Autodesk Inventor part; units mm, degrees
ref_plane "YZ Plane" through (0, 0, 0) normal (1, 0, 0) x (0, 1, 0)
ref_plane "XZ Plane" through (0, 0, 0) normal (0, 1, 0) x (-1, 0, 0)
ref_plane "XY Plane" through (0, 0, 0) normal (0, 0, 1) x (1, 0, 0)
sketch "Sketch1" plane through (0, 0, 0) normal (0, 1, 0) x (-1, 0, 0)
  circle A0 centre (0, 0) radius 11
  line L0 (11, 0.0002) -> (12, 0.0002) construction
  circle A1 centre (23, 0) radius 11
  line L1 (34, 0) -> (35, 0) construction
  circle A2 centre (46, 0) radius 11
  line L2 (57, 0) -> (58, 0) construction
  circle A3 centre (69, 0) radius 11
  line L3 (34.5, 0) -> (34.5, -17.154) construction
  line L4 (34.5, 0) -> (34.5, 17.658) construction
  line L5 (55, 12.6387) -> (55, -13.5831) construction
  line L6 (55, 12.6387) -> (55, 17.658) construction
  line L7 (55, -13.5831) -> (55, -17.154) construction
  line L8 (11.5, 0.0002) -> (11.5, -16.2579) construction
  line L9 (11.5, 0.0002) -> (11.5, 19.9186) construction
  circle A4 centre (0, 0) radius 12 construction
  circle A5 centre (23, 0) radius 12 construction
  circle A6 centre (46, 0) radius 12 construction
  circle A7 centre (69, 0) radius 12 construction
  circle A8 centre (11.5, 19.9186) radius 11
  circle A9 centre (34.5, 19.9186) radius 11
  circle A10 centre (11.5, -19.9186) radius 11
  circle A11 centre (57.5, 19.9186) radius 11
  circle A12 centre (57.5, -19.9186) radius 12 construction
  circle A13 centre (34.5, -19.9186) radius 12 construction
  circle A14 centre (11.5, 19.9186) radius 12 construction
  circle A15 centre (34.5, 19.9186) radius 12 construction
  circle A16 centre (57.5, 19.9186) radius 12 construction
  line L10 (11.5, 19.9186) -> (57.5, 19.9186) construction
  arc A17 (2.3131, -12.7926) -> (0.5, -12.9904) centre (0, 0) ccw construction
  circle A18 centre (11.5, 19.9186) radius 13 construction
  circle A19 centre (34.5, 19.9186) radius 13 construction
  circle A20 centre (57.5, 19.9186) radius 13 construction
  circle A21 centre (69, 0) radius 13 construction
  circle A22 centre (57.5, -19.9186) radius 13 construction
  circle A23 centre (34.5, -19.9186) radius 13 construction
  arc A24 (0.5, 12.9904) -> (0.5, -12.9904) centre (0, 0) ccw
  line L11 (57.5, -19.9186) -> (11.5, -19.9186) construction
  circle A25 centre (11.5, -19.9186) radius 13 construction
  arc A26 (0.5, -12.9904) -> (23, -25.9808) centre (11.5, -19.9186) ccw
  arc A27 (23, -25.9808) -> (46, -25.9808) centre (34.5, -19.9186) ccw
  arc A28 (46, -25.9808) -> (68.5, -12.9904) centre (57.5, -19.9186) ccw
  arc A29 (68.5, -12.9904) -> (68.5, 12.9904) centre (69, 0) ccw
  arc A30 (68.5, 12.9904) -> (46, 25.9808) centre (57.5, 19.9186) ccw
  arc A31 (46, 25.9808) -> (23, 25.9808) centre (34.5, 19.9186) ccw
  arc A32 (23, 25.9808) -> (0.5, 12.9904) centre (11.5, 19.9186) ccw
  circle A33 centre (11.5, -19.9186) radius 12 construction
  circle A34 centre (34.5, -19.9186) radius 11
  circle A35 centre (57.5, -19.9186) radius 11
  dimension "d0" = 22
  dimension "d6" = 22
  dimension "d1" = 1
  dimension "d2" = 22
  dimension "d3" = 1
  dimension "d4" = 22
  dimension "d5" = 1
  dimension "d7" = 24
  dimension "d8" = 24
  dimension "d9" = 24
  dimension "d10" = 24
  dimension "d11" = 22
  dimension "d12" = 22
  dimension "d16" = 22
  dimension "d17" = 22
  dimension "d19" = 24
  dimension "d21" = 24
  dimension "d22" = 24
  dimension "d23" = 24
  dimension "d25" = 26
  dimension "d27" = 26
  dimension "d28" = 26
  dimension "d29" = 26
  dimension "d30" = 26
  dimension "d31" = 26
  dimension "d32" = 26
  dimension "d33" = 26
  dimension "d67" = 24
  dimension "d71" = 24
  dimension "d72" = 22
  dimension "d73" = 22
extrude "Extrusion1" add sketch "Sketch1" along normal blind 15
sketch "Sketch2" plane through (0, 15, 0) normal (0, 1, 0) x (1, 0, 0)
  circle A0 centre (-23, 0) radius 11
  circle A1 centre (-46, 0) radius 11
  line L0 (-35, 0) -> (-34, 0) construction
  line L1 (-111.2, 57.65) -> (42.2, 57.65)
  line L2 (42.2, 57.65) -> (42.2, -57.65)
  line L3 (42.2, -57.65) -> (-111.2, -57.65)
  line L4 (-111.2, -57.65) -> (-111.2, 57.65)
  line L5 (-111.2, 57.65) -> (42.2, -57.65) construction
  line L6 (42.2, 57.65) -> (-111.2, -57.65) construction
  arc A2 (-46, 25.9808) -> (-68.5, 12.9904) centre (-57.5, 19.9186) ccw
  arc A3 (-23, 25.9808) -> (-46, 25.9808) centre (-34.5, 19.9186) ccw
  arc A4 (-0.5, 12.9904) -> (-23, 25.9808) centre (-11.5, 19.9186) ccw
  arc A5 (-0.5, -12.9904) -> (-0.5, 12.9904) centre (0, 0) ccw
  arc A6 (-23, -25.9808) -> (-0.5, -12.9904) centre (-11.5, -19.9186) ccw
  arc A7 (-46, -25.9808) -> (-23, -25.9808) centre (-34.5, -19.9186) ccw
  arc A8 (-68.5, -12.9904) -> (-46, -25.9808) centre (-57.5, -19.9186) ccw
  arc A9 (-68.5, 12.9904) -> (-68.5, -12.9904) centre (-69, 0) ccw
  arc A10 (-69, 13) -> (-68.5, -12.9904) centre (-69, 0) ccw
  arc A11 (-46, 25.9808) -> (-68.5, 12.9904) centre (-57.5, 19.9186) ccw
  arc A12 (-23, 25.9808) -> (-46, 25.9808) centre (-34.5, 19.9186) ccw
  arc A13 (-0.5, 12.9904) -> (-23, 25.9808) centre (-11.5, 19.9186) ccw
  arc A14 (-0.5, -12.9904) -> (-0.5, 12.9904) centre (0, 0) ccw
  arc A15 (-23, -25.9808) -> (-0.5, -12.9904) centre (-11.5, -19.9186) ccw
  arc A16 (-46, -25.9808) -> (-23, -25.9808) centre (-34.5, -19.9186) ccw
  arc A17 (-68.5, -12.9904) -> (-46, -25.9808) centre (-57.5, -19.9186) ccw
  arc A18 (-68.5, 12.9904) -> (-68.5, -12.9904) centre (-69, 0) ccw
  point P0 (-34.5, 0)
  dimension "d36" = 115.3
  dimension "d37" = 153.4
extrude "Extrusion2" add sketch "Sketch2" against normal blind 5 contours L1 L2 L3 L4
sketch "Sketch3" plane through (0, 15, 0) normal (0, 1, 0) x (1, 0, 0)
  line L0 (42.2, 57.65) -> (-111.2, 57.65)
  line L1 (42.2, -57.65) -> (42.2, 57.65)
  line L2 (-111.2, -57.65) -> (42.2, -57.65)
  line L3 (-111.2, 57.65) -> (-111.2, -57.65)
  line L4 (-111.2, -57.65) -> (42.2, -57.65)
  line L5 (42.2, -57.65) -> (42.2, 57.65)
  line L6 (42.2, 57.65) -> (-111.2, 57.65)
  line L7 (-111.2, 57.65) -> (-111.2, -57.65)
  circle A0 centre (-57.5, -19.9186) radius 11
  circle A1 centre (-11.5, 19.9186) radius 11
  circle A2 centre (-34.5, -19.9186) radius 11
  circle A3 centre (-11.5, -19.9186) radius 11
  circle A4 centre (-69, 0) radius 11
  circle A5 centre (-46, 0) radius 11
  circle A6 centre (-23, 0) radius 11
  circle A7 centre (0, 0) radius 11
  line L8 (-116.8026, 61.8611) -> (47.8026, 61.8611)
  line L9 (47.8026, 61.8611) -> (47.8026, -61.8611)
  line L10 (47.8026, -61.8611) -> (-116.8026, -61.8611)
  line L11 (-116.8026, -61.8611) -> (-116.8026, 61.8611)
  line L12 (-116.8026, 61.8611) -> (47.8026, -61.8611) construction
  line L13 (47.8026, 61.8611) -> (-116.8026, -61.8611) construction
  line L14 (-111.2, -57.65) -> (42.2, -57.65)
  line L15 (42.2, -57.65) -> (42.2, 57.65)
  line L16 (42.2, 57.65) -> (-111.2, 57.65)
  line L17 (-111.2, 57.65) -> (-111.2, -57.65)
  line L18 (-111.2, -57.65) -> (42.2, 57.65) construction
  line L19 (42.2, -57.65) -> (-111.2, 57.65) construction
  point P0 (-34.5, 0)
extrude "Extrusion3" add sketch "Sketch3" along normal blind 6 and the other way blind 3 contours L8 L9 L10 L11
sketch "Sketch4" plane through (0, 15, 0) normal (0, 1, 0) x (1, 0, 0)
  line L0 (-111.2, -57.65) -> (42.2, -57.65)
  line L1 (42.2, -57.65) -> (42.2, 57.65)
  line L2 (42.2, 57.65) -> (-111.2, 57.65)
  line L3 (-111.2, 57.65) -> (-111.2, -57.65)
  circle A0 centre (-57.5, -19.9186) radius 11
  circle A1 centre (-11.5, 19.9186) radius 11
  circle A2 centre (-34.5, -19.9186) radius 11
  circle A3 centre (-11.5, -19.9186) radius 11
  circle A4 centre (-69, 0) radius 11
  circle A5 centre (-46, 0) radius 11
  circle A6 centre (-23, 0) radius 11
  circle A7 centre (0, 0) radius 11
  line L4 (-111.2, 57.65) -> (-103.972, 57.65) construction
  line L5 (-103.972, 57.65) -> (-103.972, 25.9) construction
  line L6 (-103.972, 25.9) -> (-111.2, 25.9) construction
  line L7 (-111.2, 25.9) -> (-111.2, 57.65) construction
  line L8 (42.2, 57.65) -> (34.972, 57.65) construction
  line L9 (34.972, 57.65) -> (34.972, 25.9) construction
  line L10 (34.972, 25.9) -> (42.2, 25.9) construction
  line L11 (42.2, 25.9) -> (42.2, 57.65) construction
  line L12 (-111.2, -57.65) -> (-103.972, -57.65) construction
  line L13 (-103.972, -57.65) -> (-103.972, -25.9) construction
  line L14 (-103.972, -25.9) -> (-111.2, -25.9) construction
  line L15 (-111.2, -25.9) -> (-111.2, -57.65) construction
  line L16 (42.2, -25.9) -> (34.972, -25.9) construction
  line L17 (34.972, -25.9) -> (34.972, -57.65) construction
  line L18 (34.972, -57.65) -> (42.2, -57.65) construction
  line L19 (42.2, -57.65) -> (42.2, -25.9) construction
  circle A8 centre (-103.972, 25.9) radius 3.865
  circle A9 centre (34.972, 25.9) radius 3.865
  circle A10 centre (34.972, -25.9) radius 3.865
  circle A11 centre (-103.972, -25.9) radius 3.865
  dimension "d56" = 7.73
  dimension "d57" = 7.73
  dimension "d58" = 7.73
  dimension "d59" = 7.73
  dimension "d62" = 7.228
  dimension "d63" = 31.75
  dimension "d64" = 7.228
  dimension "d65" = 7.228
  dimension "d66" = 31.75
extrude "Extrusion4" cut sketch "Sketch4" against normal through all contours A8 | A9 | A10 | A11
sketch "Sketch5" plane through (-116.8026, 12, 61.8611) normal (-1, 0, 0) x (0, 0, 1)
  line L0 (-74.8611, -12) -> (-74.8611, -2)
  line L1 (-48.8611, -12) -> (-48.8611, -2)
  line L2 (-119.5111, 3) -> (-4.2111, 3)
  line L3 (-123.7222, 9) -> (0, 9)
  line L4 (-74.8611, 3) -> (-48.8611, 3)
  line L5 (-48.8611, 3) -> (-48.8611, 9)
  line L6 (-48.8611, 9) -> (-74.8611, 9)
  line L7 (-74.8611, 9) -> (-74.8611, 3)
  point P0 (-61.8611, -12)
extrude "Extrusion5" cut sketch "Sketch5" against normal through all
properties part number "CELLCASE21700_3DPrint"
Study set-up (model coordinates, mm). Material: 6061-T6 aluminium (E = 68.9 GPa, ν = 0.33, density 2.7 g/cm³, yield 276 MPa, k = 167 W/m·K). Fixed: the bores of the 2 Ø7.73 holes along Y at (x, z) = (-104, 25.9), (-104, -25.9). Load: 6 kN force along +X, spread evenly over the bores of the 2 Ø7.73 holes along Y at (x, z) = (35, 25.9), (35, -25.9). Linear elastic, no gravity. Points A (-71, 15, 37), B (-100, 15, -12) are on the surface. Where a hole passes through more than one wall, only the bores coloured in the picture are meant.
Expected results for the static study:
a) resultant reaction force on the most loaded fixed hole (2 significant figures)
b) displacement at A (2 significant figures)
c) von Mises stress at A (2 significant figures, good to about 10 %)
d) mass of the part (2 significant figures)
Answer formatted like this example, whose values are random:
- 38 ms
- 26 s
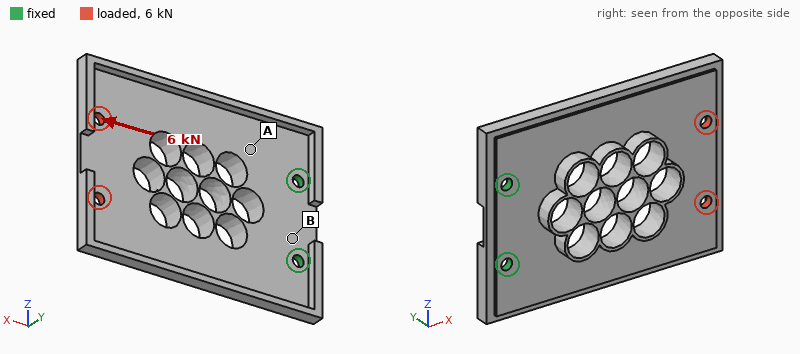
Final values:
- 3.1 kN
- 0.022 mm
- 23 MPa
- 270 g
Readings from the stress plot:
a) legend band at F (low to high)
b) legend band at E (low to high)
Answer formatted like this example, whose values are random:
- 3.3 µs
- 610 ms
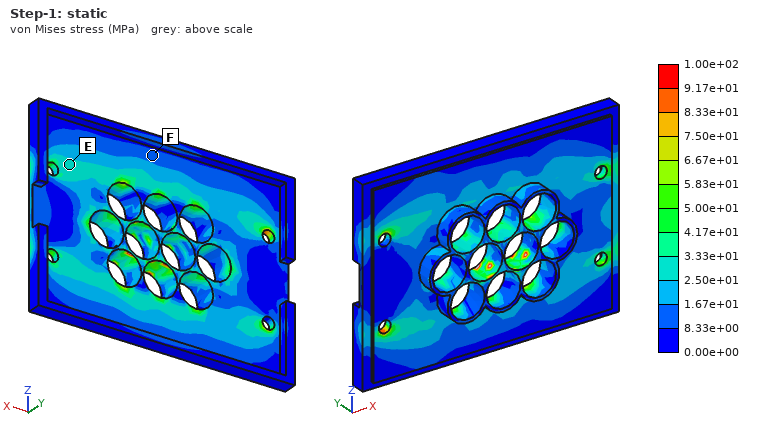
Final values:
- 8.33e+00 to 1.67e+01 MPa
- 2.50e+01 to 3.33e+01 MPa
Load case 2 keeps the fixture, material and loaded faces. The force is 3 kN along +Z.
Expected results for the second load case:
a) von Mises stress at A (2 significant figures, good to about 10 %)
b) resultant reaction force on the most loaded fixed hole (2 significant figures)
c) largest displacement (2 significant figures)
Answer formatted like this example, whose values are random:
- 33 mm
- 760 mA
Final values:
- 26 MPa
- 7.1 kN
- 0.51 mm
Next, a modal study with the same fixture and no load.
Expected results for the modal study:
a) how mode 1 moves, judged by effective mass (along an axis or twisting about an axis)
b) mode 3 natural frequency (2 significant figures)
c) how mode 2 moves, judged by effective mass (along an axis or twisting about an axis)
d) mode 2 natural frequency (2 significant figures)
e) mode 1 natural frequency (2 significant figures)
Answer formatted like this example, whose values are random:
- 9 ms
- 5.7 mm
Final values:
- along Y
- 1300 Hz
- twisting about X
- 450 Hz
- 210 Hz
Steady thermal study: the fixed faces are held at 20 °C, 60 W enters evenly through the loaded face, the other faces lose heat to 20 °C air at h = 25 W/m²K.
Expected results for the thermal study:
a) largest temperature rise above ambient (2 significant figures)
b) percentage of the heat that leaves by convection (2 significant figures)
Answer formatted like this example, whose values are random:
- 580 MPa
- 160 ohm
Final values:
- 66 K
- 61 %
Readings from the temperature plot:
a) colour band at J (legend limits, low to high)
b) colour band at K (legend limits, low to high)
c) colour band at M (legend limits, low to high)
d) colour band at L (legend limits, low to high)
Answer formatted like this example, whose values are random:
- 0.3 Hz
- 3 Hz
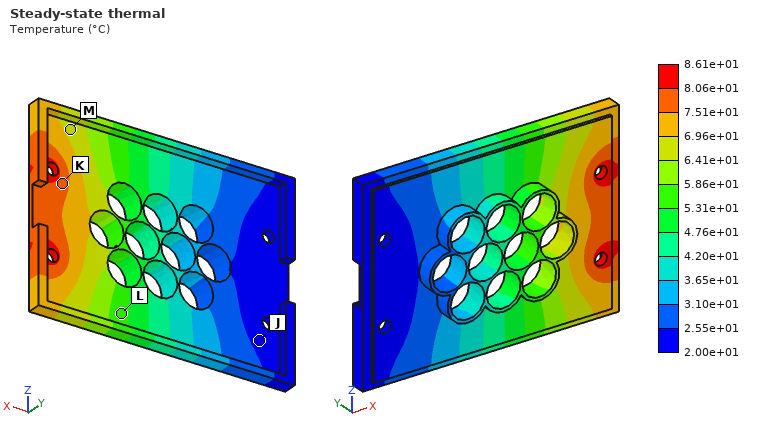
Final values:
- 2.00e+01 to 2.55e+01 °C
- 7.51e+01 to 8.06e+01 °C
- 6.41e+01 to 6.96e+01 °C
- 5.31e+01 to 5.86e+01 °C
